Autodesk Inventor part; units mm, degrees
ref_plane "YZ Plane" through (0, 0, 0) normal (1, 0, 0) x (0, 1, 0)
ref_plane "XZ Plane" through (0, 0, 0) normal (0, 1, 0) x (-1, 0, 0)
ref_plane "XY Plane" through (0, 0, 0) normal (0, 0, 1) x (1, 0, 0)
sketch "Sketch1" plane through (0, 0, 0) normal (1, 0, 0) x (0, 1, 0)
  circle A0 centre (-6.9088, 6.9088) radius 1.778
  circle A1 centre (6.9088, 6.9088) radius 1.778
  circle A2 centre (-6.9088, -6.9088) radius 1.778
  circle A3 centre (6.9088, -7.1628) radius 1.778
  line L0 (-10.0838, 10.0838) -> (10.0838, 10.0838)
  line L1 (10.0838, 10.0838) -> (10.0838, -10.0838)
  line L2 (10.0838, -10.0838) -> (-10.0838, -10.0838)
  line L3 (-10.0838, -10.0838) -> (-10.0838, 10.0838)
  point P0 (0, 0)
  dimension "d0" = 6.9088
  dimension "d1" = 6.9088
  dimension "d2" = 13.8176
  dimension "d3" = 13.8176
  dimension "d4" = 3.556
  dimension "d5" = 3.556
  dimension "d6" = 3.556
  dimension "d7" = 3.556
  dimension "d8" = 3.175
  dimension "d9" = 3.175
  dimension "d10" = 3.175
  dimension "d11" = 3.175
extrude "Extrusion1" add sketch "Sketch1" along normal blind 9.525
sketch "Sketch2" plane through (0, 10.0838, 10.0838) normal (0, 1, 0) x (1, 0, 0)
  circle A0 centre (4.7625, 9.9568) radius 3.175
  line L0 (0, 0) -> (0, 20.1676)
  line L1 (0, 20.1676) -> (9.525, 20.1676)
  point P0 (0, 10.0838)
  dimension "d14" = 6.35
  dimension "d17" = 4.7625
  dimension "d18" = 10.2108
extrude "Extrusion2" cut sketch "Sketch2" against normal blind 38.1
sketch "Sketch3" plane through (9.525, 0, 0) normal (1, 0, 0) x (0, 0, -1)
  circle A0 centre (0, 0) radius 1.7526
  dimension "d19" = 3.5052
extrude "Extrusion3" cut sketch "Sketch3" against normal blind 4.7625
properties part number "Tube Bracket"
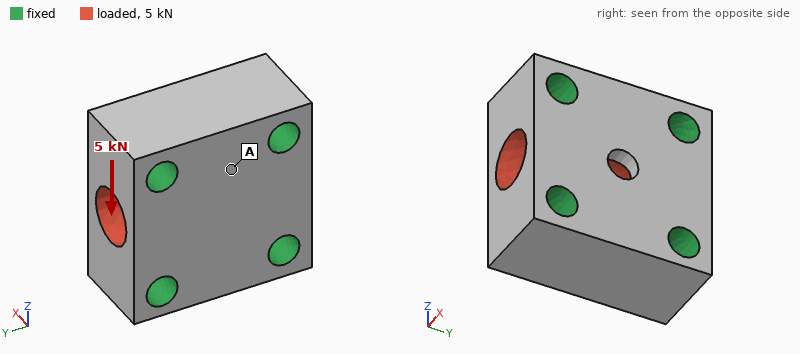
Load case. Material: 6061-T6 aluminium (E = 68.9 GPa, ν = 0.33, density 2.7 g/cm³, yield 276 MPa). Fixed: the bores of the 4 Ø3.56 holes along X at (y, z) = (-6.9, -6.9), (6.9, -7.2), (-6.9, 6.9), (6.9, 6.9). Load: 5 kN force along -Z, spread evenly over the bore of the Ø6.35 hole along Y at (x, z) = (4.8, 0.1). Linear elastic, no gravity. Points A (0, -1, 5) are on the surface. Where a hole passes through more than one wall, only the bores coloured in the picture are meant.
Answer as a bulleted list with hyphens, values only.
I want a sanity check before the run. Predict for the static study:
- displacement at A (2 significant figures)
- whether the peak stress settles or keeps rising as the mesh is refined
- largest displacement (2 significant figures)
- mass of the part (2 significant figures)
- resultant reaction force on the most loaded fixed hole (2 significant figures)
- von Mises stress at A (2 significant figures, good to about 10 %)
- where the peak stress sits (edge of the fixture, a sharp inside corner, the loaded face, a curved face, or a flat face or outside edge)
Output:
- 1.6 µm
- keeps rising
- 2.1 µm
- 7.7 g
- 1.3 kN
- 4.6 MPa
- edge of the fixture
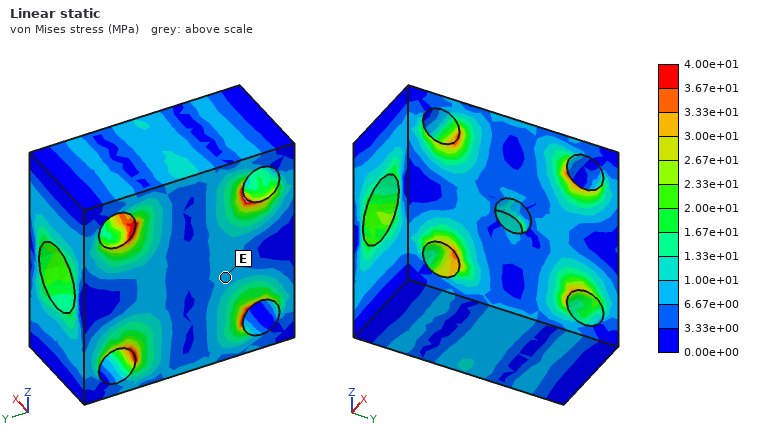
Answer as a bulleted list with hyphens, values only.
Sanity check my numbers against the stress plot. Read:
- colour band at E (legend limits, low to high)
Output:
- 6.67e+00 to 1.00e+01 MPa
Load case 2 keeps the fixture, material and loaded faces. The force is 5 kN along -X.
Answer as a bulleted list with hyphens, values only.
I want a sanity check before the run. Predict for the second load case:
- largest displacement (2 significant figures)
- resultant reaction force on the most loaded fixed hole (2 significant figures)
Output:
- 5.9 µm
- 1.3 kN
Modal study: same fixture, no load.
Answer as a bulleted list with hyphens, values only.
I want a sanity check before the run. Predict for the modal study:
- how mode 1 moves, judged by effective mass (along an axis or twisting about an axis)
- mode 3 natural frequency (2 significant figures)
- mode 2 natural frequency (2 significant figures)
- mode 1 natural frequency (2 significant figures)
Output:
- along X
- 120 kHz
- 110 kHz
- 100 kHz
